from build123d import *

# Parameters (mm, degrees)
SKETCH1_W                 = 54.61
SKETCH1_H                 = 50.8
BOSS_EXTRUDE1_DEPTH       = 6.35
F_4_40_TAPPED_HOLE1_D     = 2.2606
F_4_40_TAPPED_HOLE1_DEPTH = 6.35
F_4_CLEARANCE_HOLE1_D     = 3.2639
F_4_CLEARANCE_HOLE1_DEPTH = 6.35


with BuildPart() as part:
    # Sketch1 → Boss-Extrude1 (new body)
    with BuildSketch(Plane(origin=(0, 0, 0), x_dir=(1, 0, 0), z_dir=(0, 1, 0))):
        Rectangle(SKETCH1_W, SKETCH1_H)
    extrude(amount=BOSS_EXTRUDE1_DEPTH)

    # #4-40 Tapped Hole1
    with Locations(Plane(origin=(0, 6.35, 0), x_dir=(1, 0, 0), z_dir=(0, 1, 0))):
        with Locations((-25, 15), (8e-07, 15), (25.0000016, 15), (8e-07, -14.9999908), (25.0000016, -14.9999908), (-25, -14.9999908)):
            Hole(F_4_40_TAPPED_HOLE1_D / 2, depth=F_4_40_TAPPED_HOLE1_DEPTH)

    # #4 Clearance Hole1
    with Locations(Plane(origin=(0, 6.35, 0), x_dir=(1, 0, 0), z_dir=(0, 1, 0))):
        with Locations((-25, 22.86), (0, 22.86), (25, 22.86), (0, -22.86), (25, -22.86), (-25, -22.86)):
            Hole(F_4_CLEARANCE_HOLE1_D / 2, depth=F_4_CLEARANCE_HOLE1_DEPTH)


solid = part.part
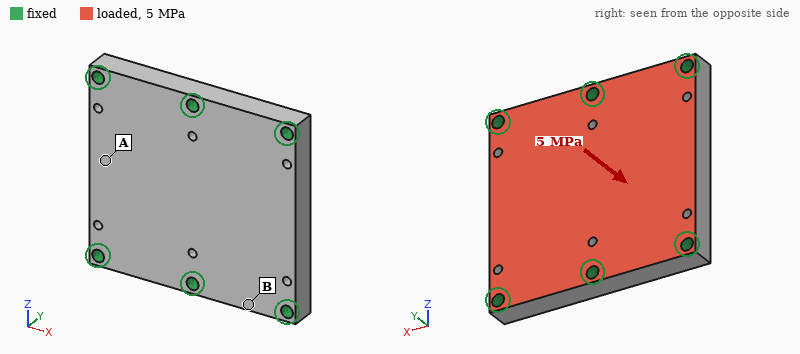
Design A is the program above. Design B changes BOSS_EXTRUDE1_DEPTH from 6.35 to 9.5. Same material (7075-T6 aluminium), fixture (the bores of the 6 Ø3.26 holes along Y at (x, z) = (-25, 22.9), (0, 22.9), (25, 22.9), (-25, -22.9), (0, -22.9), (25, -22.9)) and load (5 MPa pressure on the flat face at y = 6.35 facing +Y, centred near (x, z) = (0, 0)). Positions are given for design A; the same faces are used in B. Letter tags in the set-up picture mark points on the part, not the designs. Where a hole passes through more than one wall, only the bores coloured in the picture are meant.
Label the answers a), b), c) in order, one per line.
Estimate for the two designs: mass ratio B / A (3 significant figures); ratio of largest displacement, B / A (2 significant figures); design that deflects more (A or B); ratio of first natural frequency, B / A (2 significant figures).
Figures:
a) 1.50
b) 0.40
c) A
d) 1.3
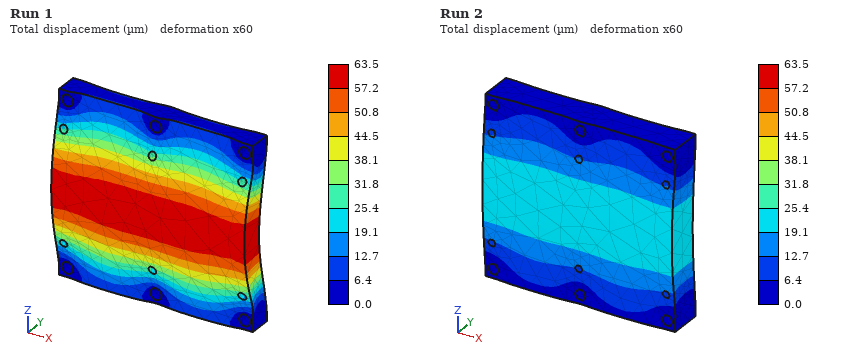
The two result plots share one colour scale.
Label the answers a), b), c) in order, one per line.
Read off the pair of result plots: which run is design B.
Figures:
a) Run 2
